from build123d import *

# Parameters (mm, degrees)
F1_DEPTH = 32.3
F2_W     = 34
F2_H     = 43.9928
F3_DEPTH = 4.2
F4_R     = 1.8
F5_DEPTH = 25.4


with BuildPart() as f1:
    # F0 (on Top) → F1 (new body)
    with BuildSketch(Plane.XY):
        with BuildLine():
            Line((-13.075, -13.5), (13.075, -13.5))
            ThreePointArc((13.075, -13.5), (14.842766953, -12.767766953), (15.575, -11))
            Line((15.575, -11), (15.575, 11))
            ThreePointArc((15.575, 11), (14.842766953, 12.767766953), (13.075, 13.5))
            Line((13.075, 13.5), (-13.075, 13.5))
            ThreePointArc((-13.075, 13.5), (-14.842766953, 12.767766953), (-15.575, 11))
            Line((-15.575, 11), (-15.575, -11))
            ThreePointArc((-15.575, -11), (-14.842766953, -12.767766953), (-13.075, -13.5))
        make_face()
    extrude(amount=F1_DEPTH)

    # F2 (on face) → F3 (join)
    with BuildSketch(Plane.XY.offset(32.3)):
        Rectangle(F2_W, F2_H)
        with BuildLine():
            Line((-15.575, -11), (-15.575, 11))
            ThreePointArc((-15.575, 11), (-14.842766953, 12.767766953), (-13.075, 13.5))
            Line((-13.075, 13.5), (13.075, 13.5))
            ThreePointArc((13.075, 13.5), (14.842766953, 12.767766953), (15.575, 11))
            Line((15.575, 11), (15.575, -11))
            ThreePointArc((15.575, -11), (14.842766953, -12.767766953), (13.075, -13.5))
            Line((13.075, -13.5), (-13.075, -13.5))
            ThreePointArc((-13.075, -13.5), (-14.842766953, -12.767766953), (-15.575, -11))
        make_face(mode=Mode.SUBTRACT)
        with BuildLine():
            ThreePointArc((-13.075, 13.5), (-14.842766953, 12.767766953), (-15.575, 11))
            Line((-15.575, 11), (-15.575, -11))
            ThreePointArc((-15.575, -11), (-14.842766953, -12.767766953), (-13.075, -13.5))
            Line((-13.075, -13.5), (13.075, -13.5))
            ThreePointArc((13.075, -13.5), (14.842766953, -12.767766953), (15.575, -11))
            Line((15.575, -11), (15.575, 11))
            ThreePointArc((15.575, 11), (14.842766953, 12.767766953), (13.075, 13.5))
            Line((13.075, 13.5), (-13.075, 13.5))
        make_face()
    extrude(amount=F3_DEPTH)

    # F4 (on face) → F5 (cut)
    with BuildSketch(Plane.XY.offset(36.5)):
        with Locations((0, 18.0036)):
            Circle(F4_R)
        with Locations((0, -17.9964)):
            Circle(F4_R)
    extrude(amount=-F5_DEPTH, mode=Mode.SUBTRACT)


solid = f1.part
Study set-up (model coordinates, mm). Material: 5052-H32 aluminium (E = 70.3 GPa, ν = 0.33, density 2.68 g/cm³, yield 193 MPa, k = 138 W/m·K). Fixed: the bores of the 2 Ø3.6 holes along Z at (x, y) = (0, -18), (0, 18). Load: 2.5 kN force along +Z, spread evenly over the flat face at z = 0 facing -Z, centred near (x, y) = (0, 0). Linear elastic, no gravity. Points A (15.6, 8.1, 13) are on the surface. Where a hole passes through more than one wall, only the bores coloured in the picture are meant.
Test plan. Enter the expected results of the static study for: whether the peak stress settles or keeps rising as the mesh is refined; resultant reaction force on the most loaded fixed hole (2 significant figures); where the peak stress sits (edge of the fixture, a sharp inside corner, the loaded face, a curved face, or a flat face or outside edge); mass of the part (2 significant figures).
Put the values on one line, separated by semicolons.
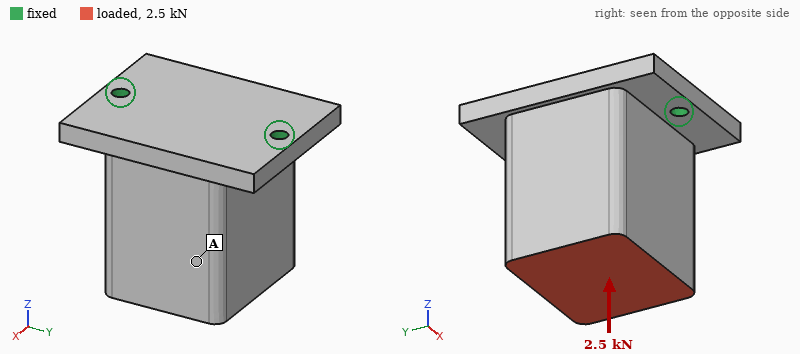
keeps rising; 1.3 kN; edge of the fixture; 89 g
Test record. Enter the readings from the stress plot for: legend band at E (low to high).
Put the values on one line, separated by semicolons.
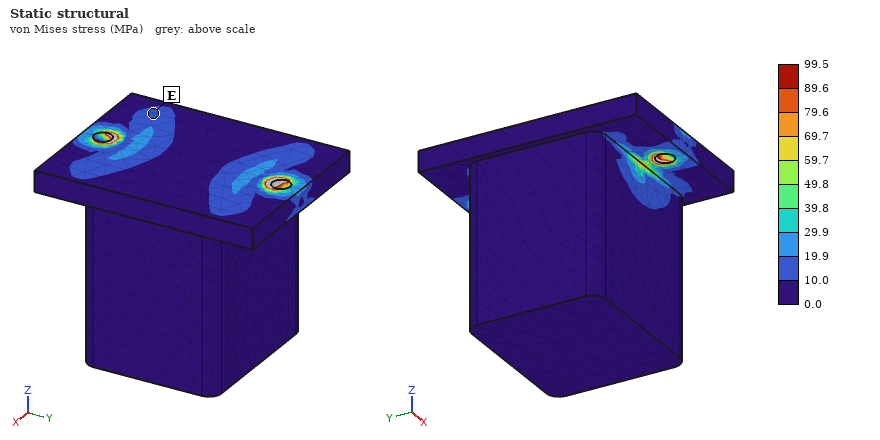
10.0 to 19.9 MPa
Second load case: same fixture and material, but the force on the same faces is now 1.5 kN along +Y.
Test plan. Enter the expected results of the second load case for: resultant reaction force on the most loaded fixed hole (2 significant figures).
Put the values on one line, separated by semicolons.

1.8 kN
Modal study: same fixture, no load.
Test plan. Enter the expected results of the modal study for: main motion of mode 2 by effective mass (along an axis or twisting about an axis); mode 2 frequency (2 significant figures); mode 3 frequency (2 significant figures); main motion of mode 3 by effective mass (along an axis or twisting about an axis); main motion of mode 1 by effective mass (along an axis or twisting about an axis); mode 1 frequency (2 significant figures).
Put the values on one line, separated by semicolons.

along Y; 6100 Hz; 8400 Hz; along Z; along X; 1800 Hz
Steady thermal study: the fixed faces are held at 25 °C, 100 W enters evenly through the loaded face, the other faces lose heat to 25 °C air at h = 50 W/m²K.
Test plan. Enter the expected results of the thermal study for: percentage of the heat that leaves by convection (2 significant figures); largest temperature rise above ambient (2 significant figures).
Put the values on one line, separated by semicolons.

12 %; 59 K
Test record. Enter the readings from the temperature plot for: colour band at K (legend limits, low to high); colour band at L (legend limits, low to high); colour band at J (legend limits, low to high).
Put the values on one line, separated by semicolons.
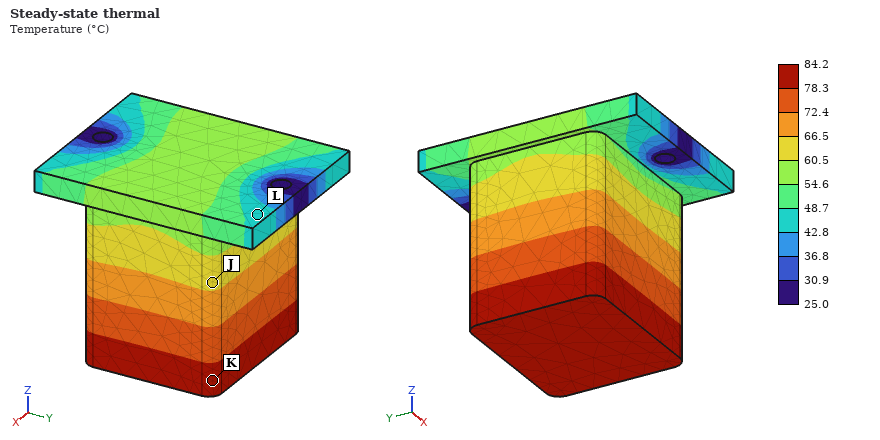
78.3 to 84.2 °C; 42.8 to 48.7 °C; 60.5 to 66.5 °C
